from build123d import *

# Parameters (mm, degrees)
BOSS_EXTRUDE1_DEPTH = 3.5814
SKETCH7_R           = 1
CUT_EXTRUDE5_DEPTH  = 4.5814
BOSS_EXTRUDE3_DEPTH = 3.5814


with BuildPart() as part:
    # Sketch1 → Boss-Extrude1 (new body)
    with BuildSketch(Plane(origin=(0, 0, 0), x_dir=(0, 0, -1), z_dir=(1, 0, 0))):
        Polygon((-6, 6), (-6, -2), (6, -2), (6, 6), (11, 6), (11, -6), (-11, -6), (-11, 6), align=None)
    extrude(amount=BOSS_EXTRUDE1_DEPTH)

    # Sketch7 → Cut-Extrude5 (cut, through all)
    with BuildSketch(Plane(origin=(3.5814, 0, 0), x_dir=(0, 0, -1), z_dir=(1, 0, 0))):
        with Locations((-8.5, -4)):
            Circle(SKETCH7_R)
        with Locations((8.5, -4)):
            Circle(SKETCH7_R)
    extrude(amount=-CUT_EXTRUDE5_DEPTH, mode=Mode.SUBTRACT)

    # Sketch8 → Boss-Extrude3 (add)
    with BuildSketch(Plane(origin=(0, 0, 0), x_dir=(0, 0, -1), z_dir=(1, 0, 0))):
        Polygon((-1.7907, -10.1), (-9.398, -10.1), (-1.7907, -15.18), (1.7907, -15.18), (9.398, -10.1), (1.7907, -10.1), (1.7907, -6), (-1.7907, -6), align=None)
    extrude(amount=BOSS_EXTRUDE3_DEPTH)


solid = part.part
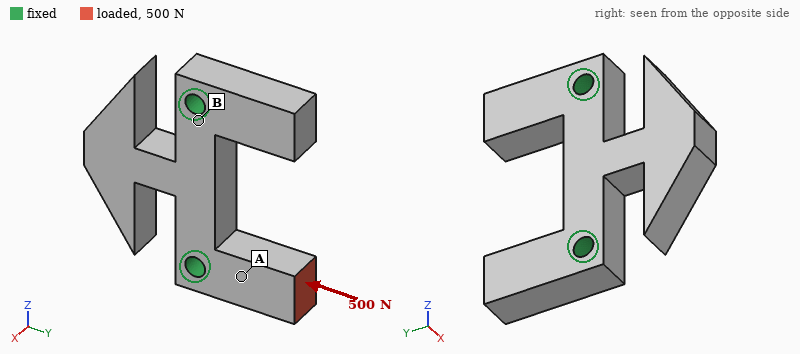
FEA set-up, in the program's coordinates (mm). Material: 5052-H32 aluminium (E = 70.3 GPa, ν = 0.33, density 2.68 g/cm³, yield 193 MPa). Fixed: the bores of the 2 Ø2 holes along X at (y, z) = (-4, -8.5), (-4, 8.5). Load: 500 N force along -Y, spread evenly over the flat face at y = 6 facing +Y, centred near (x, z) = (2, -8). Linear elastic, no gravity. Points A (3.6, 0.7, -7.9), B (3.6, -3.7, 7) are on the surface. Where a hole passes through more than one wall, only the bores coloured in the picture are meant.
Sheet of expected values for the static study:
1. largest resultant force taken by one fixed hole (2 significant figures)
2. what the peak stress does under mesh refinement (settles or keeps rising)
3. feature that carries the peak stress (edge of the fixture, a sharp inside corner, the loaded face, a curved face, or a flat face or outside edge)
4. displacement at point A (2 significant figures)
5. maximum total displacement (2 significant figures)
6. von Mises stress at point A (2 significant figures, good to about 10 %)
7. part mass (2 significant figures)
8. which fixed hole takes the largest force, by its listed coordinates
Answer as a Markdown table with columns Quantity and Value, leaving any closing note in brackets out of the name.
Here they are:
| Quantity | Value |
|---|---|
| largest resultant force taken by one fixed hole | 500 N |
| what the peak stress does under mesh refinement | keeps rising |
| feature that carries the peak stress | edge of the fixture |
| displacement at point A | 1.8 µm |
| maximum total displacement | 4.2 µm |
| von Mises stress at point A | 29 MPa |
| part mass | 2.2 g |
| which fixed hole takes the largest force, by its listed coordinates | (-4, -8.5) |
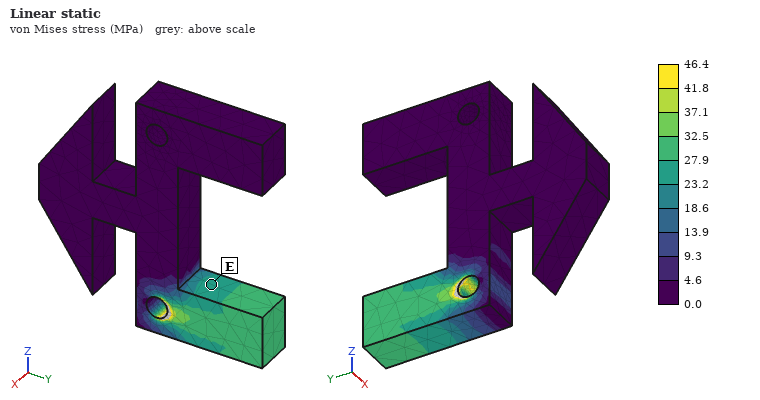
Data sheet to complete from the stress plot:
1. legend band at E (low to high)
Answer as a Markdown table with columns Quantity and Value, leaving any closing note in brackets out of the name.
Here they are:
| Quantity | Value |
|---|---|
| legend band at E | 23.2 to 27.9 MPa |
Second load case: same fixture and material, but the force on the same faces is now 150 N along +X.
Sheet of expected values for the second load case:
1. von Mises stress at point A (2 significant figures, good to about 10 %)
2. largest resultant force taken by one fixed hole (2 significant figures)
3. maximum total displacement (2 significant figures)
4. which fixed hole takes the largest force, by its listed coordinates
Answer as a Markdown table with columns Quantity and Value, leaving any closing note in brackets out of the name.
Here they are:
| Quantity | Value |
|---|---|
| von Mises stress at point A | 75 MPa |
| largest resultant force taken by one fixed hole | 160 N |
| maximum total displacement | 37 µm |
| which fixed hole takes the largest force, by its listed coordinates | (-4, -8.5) |
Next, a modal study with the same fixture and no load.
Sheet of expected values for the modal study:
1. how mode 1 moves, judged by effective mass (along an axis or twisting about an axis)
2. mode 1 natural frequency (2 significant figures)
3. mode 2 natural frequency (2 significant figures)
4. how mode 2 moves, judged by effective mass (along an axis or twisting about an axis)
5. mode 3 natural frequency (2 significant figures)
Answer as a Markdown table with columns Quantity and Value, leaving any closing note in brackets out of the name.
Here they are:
| Quantity | Value |
|---|---|
| how mode 1 moves, judged by effective mass | along X |
| mode 1 natural frequency | 9600 Hz |
| mode 2 natural frequency | 13 kHz |
| how mode 2 moves, judged by effective mass | along Z |
| mode 3 natural frequency | 17 kHz |
